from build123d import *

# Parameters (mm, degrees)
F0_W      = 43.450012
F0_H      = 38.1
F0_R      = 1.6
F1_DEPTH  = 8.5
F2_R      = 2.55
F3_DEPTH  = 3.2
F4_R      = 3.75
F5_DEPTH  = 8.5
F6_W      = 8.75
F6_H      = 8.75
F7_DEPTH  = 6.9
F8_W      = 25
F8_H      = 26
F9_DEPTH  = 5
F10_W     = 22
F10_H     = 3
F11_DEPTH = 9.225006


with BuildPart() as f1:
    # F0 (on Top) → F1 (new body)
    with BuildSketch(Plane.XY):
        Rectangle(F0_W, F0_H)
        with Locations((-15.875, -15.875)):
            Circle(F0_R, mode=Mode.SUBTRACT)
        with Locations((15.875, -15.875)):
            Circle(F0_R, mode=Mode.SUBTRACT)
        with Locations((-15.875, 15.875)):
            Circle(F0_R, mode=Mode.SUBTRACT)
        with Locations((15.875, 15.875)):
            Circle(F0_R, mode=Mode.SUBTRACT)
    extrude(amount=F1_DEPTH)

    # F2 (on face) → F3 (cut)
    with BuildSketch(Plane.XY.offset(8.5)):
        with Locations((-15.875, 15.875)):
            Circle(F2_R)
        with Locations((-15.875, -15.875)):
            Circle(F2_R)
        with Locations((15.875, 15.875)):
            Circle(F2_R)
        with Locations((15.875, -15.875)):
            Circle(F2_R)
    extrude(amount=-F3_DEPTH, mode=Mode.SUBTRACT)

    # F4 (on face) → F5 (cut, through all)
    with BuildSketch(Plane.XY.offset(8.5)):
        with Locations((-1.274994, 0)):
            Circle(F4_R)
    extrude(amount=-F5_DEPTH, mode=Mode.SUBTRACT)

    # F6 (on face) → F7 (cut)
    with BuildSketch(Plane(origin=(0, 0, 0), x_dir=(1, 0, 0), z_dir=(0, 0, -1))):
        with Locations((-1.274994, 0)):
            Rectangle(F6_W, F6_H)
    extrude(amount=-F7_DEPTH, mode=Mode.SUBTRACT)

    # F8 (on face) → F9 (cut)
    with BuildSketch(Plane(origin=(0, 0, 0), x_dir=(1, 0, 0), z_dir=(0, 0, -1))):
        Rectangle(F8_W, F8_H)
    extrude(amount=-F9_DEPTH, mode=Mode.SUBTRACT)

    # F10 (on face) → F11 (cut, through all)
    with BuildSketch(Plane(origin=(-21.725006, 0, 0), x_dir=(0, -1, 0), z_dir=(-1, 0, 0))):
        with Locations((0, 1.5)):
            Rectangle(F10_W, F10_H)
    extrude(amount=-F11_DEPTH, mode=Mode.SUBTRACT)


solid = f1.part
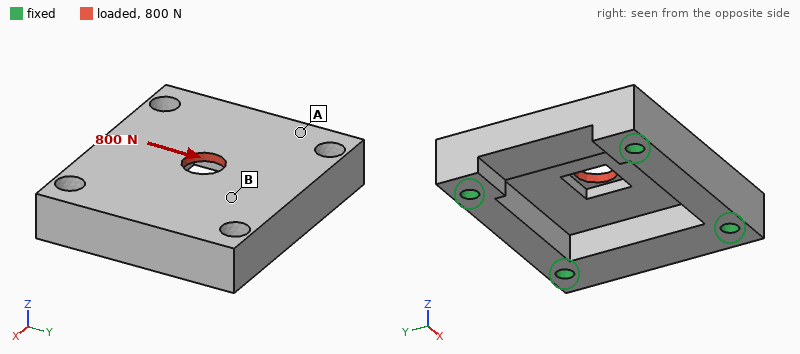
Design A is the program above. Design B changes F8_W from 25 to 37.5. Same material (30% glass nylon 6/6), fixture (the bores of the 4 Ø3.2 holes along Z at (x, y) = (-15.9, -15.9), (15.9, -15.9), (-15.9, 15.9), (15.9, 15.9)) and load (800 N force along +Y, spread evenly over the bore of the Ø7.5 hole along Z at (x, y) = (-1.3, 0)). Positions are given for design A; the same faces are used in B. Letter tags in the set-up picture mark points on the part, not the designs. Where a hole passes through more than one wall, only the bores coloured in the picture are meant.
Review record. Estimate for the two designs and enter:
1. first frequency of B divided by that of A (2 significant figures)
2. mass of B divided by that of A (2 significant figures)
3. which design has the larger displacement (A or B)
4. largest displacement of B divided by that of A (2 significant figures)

0.84
0.87
B
1.1
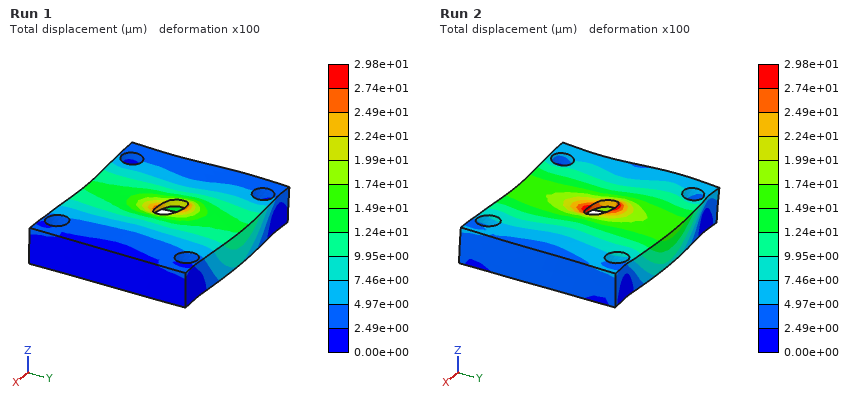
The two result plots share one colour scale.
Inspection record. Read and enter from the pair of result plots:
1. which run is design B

Run 2
